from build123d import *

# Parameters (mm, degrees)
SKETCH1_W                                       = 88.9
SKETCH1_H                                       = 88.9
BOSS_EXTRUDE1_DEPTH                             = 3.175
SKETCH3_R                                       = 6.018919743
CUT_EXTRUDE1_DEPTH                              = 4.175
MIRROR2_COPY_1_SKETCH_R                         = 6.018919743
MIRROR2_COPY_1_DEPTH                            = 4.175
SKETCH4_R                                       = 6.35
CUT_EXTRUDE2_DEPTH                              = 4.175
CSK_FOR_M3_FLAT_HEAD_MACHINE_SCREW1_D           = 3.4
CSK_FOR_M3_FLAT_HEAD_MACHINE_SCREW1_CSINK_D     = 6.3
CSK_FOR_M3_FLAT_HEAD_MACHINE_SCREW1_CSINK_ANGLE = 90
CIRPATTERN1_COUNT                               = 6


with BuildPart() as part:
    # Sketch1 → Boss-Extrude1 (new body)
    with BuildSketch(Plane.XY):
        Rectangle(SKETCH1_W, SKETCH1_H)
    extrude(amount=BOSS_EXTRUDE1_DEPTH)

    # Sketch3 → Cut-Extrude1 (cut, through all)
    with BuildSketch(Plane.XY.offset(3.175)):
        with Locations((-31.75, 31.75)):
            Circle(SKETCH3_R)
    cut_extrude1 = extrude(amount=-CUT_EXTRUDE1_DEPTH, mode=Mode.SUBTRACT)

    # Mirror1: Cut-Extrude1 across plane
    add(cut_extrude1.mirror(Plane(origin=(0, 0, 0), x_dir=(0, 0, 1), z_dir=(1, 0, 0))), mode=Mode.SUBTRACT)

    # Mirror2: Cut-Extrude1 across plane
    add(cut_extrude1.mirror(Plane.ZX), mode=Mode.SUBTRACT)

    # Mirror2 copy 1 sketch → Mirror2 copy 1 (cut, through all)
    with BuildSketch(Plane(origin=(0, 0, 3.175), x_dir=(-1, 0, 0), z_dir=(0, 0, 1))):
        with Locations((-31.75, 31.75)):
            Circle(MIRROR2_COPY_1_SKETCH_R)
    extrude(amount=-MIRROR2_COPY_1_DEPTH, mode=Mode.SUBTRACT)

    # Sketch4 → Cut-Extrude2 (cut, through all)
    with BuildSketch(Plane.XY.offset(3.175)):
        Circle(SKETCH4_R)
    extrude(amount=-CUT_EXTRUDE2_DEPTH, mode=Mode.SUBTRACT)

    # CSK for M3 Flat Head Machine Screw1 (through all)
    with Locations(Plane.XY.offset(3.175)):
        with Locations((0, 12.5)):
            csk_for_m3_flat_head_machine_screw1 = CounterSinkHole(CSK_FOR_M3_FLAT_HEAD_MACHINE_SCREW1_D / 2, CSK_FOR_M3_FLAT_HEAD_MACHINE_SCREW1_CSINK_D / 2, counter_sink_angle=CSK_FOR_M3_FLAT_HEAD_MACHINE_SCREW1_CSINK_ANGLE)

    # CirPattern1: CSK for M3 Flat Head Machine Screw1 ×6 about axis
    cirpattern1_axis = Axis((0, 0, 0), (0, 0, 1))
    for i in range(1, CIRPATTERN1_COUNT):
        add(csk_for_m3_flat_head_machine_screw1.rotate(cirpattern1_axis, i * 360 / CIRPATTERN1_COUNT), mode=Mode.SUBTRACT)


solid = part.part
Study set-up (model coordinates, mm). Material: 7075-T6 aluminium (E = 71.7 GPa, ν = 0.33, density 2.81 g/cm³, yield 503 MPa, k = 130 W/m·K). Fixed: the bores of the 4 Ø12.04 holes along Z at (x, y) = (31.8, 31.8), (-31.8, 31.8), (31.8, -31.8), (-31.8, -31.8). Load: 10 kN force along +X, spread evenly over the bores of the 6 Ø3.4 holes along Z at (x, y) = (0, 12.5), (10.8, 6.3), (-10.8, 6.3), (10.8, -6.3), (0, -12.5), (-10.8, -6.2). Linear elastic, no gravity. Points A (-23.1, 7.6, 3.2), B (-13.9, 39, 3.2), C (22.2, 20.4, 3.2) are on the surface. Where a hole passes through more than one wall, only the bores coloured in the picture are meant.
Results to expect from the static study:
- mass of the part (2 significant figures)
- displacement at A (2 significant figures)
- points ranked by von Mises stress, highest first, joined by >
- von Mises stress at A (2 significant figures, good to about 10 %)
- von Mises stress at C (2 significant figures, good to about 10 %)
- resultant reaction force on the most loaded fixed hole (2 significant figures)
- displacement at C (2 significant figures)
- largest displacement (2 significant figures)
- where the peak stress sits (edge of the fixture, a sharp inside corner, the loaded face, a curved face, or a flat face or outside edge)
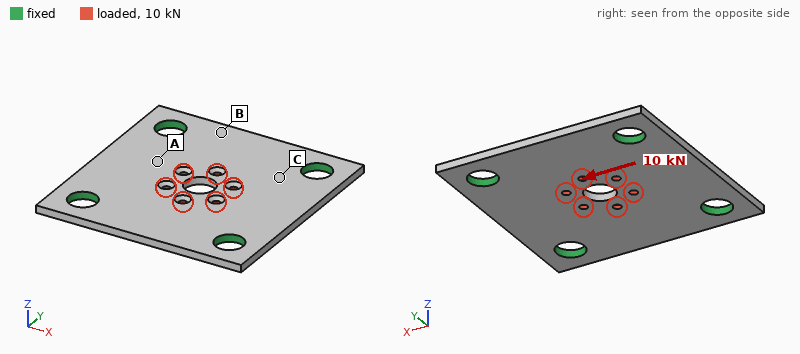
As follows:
65 g
21 µm
C > A > B
24 MPa
41 MPa
2.8 kN
9.5 µm
29 µm
the loaded face
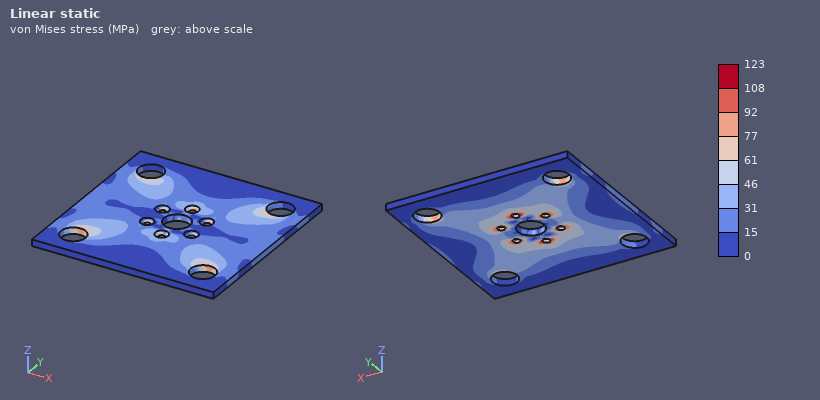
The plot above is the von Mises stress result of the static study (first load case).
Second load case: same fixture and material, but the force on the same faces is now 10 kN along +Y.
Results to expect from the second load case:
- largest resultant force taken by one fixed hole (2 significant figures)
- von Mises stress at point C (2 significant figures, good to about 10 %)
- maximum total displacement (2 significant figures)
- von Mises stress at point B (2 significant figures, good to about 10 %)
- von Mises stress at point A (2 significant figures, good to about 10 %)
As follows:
2.8 kN
40 MPa
30 µm
19 MPa
21 MPa
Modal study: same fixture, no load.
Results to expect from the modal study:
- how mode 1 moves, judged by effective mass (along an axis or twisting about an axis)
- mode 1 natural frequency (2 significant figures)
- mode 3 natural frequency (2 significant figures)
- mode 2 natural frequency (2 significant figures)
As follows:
along Z
3800 Hz
5700 Hz
5700 Hz
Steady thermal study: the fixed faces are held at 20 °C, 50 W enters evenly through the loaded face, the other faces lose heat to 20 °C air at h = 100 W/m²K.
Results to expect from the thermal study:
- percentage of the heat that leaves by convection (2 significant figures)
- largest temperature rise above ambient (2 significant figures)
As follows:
26 %
29 K
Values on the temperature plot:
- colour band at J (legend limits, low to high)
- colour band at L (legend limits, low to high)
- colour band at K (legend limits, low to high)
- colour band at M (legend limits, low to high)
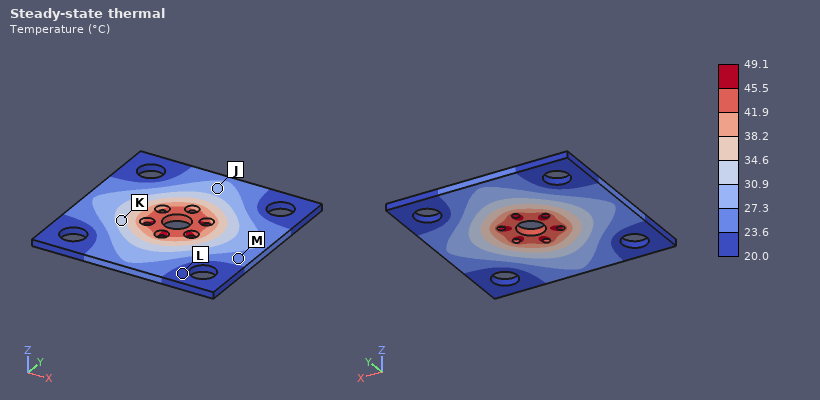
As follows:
27.3 to 30.9 °C
20.0 to 23.6 °C
30.9 to 34.6 °C
23.6 to 27.3 °C
